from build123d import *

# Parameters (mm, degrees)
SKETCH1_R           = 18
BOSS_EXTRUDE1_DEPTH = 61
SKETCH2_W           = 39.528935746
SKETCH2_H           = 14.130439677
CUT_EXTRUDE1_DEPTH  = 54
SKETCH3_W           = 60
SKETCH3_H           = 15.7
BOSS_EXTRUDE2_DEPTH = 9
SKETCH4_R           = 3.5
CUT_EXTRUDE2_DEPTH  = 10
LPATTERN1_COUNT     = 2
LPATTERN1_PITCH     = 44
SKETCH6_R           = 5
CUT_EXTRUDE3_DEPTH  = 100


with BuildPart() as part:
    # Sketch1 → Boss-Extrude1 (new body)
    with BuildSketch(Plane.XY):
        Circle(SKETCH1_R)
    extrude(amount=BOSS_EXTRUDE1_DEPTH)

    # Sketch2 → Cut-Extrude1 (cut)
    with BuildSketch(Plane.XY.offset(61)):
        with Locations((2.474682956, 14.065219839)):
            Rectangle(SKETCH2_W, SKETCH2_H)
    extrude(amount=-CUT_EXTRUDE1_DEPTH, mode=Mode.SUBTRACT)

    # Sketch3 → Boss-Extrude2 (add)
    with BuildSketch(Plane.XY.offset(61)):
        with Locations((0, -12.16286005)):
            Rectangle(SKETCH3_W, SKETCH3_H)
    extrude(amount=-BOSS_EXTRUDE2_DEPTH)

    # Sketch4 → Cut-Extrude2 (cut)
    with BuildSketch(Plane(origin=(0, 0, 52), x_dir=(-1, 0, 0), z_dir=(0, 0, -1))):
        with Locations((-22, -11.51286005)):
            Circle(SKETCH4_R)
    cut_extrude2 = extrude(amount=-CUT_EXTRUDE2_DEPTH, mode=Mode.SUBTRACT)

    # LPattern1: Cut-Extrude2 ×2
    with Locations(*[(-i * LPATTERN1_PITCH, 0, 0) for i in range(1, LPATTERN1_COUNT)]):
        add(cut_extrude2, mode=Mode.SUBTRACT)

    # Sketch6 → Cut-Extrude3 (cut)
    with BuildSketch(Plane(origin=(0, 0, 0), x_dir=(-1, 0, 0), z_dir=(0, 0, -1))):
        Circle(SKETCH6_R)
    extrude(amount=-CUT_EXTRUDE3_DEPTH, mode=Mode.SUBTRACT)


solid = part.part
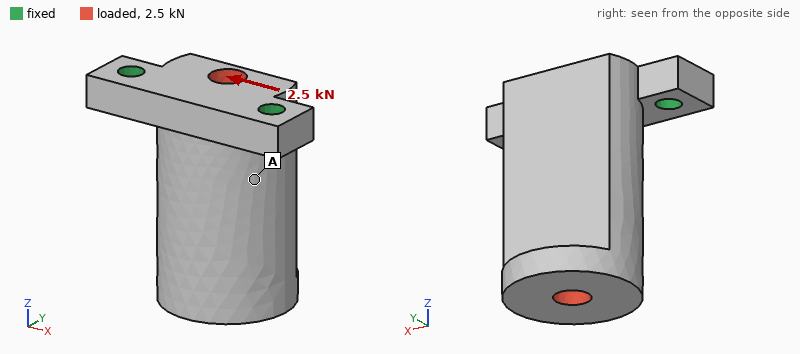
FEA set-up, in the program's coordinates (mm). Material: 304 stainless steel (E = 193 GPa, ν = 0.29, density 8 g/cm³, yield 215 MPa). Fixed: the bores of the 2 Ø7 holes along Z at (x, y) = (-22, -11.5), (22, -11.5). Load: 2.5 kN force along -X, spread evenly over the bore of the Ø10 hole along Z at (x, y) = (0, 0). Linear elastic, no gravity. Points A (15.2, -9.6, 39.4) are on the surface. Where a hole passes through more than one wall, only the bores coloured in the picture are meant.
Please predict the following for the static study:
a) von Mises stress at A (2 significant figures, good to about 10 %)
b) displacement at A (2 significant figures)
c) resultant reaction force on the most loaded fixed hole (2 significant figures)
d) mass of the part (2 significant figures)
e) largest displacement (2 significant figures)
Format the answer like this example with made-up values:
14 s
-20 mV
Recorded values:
9.5 MPa
4.5 µm
2.3 kN
380 g
15 µm
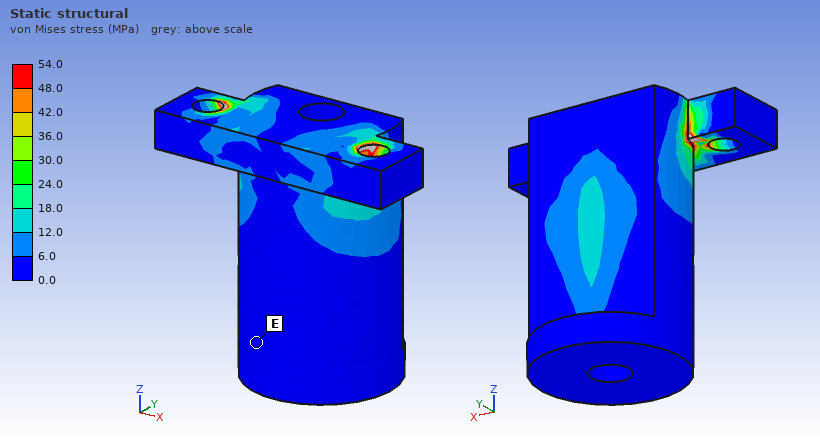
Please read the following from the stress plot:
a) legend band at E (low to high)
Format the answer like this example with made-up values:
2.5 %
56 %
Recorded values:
0.0 to 6.0 MPa
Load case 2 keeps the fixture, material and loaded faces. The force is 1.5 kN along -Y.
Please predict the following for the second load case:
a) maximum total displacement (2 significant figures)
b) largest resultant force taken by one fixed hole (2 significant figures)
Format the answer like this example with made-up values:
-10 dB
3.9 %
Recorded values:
57 µm
780 N
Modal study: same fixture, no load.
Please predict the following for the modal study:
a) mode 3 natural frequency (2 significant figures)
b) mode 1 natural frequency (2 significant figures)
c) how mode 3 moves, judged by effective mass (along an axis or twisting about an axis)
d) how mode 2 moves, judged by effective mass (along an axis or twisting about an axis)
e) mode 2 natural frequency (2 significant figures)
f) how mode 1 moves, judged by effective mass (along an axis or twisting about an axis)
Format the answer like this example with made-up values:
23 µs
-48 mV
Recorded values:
9400 Hz
1700 Hz
along Z
along X
4200 Hz
along Y
